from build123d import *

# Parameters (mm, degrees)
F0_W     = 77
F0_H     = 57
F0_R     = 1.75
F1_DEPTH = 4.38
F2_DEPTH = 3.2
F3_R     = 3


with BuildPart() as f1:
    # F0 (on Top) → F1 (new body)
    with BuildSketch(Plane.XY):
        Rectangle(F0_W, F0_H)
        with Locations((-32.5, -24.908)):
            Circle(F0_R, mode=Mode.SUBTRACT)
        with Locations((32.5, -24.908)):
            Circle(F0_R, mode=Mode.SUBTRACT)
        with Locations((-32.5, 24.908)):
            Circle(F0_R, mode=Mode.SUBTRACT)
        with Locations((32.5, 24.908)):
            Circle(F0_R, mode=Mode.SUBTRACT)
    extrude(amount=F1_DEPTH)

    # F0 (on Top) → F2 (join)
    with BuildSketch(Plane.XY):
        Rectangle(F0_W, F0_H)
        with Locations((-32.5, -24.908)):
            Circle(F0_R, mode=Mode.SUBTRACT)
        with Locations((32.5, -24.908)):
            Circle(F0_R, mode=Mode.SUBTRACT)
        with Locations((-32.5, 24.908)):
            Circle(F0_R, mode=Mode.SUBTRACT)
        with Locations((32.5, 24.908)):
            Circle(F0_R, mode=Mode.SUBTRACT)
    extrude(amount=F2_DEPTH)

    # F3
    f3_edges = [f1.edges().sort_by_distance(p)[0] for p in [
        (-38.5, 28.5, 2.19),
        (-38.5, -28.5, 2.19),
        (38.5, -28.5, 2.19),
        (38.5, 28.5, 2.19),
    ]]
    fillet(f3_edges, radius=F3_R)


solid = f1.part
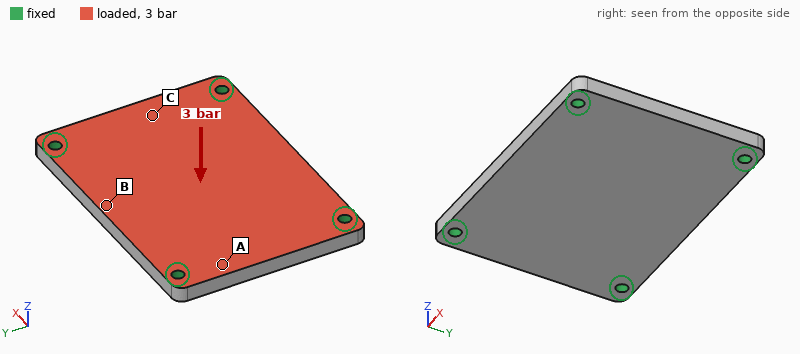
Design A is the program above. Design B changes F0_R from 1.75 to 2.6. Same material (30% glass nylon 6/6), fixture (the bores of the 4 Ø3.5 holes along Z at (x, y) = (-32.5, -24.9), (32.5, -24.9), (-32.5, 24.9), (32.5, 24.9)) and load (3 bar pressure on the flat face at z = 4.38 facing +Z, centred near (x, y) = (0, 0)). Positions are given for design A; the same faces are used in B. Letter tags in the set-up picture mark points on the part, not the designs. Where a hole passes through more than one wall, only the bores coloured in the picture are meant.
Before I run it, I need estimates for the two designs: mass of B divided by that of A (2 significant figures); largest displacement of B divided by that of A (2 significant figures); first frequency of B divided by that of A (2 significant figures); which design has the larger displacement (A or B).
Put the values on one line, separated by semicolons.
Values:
0.99; 0.86; 1.1; A
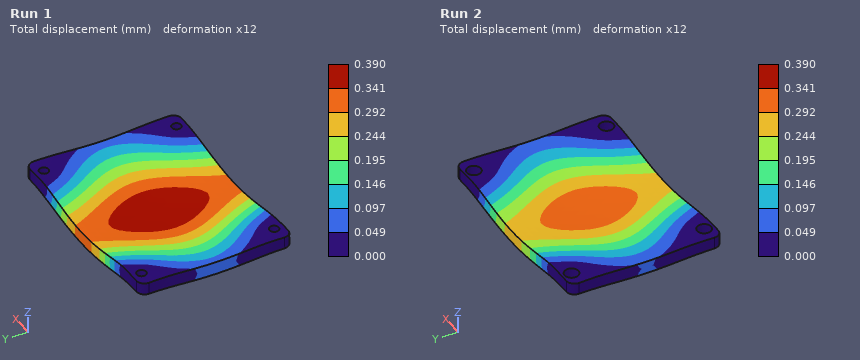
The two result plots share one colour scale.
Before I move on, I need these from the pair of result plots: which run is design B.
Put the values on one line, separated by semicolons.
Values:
Run 2
